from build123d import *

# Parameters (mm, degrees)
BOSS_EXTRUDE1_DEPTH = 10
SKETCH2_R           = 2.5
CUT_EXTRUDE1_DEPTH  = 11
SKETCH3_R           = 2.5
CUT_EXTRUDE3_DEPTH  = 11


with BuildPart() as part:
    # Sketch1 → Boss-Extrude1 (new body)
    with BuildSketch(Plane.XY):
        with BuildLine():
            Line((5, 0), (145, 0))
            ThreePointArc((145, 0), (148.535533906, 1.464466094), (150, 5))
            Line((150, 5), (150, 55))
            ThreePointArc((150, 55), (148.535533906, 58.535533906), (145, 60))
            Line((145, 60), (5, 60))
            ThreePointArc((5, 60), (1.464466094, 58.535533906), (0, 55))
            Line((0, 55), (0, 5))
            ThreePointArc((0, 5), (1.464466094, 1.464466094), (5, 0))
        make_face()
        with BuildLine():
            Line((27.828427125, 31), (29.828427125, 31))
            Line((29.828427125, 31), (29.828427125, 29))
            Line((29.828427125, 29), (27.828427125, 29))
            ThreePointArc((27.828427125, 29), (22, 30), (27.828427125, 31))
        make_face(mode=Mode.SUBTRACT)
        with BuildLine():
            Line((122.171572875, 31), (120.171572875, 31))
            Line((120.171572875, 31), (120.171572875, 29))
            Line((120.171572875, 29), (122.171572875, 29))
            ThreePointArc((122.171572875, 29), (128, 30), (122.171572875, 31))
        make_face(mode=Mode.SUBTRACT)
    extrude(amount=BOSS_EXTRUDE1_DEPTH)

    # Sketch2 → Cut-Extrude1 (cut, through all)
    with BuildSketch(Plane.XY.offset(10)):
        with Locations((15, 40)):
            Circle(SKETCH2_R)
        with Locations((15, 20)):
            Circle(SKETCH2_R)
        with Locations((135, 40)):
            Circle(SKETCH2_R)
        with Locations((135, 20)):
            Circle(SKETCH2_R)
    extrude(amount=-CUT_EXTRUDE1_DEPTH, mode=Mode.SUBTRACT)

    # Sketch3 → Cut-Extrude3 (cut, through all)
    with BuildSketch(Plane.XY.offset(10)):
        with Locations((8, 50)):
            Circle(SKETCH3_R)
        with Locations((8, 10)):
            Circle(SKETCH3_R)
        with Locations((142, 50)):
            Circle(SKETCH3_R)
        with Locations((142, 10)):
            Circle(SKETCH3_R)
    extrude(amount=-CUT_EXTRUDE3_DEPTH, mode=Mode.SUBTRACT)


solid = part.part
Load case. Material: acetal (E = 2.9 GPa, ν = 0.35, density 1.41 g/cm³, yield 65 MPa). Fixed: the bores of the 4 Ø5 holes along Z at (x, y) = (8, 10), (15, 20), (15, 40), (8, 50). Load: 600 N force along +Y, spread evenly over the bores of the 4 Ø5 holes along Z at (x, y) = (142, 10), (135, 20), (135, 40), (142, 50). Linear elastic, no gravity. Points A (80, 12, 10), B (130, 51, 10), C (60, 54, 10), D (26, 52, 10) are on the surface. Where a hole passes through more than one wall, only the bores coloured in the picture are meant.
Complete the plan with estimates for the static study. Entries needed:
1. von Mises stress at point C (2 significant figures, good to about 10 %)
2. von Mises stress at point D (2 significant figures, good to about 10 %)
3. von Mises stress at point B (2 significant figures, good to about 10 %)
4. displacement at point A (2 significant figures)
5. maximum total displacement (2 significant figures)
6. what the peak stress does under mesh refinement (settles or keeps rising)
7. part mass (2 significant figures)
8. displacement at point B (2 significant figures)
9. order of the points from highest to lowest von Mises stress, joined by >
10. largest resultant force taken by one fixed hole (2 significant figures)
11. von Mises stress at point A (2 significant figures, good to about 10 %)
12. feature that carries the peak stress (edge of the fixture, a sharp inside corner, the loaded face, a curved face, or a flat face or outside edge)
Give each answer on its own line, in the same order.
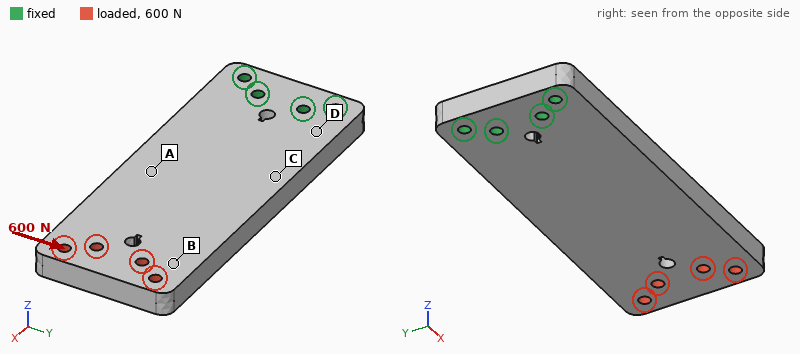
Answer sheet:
6.4 MPa
8.3 MPa
1.6 MPa
0.44 mm
1.2 mm
keeps rising
120 g
0.96 mm
D > C > A > B
1.3 kN
3.9 MPa
edge of the fixture
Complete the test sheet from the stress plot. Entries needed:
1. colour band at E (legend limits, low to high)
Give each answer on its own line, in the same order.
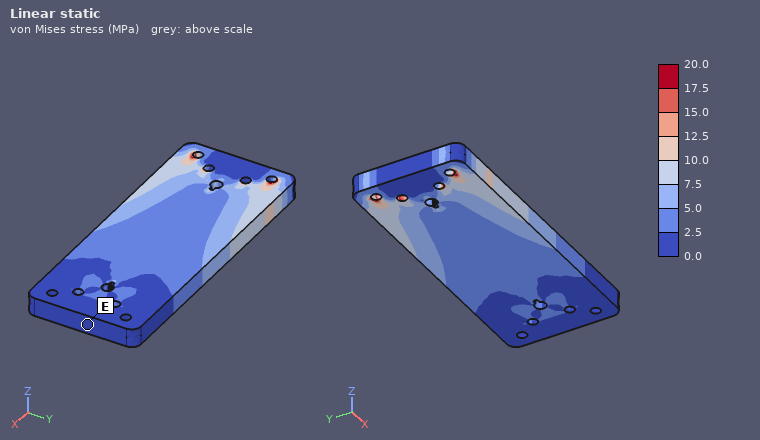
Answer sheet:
0.0 to 2.5 MPa
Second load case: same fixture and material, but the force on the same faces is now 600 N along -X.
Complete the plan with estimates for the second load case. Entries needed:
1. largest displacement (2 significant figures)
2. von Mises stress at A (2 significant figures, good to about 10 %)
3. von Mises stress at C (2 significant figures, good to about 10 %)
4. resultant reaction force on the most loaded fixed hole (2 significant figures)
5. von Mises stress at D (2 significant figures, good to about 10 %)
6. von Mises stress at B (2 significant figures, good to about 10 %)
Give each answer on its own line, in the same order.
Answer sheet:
49 µm
1.0 MPa
0.99 MPa
170 N
0.91 MPa
0.98 MPa
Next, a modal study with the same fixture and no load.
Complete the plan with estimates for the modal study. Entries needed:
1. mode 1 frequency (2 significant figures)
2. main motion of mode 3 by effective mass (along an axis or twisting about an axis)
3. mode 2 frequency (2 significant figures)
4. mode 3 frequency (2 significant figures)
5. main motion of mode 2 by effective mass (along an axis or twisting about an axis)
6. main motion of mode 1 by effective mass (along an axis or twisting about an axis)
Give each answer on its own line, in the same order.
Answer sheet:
130 Hz
along Y
550 Hz
610 Hz
twisting about X
along Z
